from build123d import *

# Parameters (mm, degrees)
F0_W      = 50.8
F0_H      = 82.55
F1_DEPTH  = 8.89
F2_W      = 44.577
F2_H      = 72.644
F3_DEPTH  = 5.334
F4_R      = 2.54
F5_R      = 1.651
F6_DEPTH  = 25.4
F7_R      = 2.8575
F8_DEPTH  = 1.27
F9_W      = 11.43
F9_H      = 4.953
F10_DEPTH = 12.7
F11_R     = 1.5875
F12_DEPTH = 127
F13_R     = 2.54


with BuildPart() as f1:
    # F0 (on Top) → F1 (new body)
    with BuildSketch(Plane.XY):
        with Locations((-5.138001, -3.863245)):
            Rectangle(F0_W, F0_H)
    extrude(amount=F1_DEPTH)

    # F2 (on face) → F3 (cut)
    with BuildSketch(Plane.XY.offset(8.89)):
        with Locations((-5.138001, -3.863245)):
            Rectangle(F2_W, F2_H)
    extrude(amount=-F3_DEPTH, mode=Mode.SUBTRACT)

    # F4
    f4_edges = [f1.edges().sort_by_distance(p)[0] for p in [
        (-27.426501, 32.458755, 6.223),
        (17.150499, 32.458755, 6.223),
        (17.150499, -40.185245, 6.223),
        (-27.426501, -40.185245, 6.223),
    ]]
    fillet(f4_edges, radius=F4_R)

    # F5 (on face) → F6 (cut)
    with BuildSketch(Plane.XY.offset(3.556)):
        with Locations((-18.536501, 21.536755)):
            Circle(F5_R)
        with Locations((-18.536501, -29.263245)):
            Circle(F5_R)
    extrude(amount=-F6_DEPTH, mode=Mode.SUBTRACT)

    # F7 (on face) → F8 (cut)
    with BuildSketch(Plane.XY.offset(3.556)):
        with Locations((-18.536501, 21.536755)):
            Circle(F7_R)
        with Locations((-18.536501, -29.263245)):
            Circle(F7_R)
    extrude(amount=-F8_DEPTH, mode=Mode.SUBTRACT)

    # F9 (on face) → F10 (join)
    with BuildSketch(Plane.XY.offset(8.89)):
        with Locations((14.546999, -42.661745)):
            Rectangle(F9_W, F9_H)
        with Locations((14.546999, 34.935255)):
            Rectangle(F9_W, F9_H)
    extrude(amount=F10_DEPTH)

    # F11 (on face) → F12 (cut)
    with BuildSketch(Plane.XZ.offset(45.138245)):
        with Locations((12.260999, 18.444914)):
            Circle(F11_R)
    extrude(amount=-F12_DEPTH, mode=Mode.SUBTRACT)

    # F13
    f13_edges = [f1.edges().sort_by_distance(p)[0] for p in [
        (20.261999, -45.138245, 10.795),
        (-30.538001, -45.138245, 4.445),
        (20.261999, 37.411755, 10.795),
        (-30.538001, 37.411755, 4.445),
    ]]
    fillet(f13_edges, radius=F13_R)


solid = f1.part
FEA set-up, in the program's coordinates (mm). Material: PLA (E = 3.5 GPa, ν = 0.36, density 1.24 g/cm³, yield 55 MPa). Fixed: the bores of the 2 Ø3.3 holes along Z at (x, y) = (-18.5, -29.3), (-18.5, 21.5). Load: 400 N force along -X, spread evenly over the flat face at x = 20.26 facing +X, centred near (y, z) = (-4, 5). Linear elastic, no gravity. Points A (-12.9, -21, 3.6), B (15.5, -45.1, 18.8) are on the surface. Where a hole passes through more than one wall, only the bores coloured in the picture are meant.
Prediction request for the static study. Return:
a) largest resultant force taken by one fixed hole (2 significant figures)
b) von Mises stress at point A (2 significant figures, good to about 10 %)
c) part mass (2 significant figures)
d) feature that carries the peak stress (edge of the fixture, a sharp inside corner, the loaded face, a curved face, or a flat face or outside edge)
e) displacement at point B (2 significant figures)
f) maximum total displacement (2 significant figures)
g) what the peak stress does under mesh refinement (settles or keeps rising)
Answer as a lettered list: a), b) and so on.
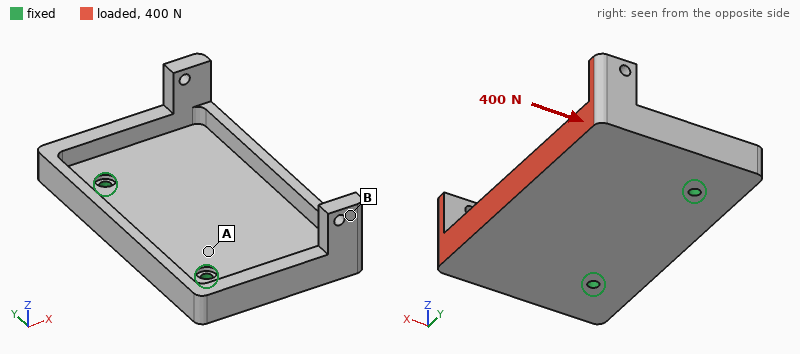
a) 200 N
b) 5.8 MPa
c) 26 g
d) edge of the fixture
e) 0.98 mm
f) 1.2 mm
g) keeps rising
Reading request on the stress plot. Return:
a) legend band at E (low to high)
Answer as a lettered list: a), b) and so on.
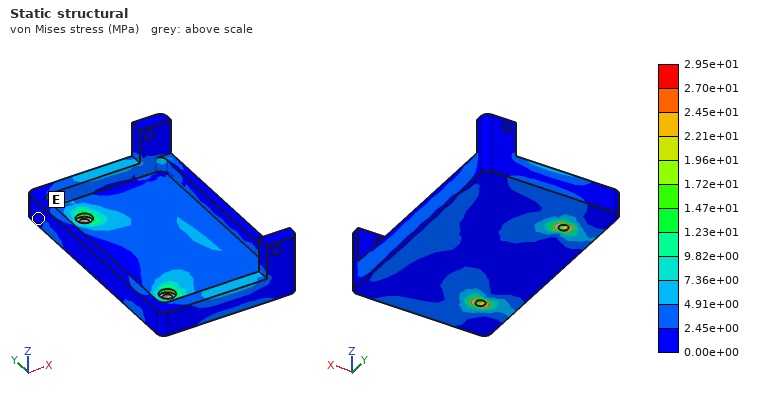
a) 0.00e+00 to 2.45e+00 MPa
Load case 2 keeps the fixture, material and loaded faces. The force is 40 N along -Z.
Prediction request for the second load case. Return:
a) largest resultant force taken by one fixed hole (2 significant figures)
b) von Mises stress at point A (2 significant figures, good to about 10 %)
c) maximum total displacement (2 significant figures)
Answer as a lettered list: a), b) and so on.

a) 20 N
b) 4.9 MPa
c) 1.0 mm
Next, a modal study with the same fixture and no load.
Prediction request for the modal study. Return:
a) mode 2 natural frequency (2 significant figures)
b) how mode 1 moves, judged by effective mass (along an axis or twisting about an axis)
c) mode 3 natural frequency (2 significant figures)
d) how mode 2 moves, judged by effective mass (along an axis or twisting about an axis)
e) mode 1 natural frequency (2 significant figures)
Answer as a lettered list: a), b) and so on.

a) 590 Hz
b) along Z
c) 1400 Hz
d) twisting about X
e) 370 Hz
